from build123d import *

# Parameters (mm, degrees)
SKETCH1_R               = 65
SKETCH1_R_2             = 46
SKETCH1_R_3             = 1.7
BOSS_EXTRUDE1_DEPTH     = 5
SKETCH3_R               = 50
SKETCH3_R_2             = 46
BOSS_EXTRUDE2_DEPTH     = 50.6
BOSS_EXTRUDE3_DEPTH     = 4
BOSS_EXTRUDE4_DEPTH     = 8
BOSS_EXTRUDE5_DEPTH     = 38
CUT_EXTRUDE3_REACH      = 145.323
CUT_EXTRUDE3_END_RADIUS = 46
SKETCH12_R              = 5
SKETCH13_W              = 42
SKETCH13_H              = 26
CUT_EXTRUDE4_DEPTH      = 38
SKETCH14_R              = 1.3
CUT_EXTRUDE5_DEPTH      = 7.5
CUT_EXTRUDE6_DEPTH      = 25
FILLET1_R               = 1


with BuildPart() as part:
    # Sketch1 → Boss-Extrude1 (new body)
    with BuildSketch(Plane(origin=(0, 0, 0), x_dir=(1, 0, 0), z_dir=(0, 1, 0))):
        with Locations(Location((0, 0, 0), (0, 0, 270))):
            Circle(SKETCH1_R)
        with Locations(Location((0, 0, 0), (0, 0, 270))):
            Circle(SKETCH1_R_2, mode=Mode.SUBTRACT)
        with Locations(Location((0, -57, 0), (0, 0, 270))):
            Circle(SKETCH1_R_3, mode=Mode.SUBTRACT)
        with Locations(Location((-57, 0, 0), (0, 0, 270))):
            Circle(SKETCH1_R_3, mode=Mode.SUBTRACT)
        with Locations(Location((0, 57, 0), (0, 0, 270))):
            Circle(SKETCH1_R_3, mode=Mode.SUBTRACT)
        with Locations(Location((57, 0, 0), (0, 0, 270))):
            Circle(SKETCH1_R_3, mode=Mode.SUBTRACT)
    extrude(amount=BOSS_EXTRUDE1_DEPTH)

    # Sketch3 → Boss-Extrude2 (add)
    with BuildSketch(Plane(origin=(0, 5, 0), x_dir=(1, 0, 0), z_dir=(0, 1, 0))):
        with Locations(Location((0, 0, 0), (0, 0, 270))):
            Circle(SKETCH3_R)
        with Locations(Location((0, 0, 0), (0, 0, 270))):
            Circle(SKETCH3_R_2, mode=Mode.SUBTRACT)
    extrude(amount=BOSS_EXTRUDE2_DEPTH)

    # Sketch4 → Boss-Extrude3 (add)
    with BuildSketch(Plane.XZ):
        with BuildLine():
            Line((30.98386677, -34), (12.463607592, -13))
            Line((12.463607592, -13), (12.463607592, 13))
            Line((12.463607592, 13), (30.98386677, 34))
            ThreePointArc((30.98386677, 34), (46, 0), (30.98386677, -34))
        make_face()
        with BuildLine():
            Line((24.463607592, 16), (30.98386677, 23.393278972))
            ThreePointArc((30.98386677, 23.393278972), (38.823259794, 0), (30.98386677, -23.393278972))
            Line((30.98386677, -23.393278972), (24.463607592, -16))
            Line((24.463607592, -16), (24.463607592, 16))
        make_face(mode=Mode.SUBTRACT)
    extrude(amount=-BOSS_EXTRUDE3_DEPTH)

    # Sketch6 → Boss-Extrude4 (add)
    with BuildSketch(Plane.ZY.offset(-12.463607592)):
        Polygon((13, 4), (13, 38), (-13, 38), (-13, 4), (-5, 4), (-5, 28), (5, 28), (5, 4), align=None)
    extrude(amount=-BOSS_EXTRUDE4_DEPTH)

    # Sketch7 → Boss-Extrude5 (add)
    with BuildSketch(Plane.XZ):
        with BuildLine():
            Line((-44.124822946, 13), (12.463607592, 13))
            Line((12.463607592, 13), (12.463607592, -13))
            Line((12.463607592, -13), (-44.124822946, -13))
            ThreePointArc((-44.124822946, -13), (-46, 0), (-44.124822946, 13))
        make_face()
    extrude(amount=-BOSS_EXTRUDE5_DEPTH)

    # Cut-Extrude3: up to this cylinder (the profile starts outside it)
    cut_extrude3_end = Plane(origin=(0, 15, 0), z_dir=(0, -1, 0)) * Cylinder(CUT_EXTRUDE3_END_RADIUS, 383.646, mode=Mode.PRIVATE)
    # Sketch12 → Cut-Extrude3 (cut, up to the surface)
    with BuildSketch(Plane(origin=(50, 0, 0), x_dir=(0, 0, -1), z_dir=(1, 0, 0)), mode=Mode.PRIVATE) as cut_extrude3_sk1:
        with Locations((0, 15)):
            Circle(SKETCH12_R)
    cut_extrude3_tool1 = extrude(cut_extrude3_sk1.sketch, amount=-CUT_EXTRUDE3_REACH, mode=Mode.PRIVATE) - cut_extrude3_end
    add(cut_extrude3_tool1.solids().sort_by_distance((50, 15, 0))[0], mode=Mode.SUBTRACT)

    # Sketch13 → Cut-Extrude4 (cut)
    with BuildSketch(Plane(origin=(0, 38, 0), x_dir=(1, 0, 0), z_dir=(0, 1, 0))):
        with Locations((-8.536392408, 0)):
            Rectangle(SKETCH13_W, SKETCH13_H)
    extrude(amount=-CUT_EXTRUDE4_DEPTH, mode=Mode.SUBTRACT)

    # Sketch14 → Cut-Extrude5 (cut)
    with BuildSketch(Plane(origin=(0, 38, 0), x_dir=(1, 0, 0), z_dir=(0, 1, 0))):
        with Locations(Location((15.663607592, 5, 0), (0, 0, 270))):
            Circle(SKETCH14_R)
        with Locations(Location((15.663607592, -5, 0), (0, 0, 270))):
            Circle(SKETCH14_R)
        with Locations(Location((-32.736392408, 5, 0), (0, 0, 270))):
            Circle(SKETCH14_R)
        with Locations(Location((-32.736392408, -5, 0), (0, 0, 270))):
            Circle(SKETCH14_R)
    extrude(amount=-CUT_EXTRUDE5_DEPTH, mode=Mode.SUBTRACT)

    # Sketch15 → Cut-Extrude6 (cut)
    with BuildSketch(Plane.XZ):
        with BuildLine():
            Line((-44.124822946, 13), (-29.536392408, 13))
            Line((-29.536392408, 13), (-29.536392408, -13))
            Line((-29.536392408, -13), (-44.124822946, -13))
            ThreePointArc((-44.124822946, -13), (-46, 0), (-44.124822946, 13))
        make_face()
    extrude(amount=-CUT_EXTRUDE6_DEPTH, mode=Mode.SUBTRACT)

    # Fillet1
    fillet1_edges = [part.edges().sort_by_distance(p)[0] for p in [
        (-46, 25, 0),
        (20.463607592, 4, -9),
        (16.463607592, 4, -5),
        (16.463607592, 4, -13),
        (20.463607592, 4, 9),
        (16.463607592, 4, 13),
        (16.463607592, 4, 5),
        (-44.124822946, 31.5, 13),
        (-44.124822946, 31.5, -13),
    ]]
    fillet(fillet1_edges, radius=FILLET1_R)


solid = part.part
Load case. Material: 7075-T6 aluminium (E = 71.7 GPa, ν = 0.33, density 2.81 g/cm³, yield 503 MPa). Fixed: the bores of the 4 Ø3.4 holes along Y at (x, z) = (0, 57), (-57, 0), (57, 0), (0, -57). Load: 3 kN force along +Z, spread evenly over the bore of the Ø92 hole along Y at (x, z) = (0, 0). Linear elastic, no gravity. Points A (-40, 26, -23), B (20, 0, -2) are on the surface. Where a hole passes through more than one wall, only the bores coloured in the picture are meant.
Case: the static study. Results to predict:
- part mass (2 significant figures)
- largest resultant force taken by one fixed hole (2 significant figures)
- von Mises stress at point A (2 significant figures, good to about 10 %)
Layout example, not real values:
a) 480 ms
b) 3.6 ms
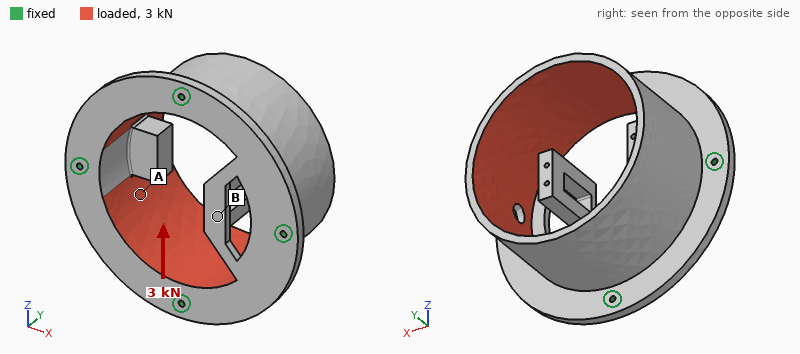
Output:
a) 300 g
b) 1.0 kN
c) 3.9 MPa
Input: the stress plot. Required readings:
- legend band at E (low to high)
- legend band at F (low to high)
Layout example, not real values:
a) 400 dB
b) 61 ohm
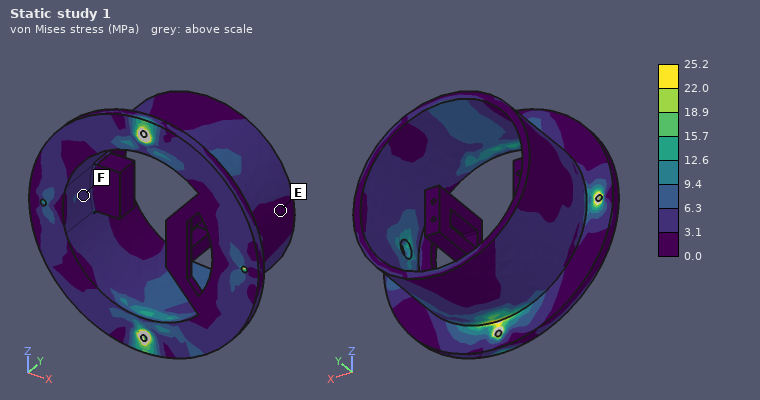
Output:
a) 0.0 to 3.1 MPa
b) 3.1 to 6.3 MPa
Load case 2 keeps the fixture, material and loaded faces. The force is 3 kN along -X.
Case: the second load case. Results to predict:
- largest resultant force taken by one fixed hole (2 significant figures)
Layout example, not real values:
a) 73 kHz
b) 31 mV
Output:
a) 990 N
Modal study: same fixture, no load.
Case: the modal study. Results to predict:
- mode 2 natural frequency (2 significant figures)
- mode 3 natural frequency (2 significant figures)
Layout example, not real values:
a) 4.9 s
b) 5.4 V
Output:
a) 1800 Hz
b) 2300 Hz
